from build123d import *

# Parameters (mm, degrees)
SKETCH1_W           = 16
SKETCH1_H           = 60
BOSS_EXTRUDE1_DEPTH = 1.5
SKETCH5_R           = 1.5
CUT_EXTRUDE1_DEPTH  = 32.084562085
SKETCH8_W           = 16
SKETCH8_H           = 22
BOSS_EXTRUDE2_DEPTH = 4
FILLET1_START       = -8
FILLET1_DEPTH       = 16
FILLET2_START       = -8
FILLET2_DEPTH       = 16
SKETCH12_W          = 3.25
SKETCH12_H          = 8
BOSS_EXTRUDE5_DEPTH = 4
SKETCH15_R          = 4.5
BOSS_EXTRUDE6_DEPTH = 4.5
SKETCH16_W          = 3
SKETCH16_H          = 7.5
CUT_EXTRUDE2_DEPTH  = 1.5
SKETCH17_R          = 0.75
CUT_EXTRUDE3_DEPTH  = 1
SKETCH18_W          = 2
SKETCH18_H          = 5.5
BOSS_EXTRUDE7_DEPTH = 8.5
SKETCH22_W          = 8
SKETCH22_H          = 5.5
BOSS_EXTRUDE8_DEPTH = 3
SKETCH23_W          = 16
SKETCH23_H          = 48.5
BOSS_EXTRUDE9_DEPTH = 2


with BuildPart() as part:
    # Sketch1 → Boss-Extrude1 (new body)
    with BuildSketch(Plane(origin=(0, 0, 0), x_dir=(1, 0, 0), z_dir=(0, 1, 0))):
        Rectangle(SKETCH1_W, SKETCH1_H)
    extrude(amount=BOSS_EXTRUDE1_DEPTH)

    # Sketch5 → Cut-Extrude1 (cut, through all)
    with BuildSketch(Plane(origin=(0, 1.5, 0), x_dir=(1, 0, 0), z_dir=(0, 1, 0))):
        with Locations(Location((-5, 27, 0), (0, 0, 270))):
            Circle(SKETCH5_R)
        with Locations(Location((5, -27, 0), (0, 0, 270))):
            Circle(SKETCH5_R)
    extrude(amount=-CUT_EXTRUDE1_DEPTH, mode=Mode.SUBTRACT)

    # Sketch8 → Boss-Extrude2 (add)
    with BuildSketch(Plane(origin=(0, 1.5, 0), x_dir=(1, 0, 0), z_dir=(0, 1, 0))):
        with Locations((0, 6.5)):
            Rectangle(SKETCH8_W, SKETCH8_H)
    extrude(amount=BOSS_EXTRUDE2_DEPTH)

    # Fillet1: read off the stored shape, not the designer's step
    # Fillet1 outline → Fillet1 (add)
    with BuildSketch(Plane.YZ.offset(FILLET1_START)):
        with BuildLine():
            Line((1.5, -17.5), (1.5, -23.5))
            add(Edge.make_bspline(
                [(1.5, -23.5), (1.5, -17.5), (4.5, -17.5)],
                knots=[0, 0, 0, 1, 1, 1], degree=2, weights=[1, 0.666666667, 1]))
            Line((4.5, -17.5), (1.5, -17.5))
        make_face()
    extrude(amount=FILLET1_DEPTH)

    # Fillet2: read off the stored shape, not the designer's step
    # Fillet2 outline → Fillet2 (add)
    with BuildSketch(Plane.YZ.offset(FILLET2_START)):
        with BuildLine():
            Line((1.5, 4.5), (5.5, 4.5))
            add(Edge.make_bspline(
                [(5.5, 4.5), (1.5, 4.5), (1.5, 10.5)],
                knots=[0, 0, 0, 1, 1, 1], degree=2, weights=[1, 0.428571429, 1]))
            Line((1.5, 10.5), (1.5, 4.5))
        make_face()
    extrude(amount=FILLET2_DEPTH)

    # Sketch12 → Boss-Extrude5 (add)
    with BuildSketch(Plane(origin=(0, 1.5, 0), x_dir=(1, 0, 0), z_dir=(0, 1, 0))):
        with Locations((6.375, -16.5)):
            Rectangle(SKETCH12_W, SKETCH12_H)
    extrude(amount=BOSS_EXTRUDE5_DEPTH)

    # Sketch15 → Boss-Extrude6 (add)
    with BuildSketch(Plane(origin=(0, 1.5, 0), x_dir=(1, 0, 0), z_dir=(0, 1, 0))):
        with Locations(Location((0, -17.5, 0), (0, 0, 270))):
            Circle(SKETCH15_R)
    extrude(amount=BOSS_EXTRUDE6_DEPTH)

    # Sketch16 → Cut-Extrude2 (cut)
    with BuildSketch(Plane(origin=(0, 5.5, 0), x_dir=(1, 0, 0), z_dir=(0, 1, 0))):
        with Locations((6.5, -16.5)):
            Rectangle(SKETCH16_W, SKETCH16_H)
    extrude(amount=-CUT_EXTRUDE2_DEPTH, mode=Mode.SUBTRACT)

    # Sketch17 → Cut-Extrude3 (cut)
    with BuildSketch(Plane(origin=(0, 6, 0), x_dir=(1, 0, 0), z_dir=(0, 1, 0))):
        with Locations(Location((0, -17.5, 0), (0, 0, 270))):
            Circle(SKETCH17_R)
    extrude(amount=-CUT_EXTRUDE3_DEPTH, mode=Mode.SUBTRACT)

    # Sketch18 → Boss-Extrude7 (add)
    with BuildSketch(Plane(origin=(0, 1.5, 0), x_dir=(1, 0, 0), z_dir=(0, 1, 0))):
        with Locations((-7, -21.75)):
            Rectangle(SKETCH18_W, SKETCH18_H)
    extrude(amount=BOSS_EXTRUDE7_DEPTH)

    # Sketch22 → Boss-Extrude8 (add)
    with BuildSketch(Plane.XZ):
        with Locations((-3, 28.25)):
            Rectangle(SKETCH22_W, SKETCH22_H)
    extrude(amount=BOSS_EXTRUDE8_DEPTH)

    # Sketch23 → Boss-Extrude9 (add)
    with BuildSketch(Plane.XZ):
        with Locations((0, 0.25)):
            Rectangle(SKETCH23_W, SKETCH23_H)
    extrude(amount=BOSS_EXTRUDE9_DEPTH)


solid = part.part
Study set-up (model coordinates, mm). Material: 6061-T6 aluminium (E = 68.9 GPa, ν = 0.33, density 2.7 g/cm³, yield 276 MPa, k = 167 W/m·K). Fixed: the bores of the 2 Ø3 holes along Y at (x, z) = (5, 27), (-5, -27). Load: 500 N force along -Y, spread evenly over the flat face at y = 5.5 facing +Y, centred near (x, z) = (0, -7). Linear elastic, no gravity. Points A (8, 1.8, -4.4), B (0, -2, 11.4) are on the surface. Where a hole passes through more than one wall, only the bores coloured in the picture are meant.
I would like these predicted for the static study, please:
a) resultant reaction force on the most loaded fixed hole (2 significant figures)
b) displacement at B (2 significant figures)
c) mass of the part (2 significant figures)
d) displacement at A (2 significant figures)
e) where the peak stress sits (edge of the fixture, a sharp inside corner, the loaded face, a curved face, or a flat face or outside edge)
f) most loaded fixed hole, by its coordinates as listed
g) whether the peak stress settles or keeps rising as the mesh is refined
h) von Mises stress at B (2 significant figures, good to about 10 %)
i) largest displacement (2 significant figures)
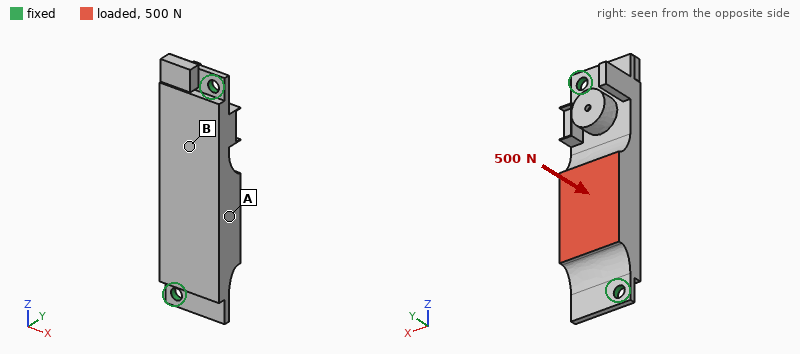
340 N
63 µm
14 g
88 µm
edge of the fixture
(-5, -27)
keeps rising
61 MPa
91 µm
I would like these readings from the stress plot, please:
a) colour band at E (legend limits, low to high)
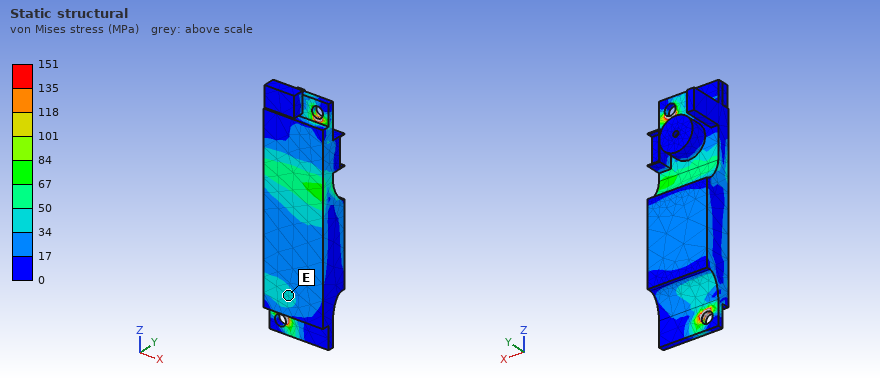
34 to 50 MPa
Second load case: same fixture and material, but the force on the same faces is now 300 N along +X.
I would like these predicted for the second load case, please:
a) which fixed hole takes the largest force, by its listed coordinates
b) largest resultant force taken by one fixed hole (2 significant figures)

(-5, -27)
190 N
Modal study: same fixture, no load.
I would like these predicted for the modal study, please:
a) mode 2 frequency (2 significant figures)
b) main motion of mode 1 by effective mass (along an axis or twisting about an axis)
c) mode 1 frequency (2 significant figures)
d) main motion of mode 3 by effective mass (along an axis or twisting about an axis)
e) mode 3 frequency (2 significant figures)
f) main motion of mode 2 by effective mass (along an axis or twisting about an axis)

4200 Hz
twisting about Z
4000 Hz
along X
9500 Hz
along Y
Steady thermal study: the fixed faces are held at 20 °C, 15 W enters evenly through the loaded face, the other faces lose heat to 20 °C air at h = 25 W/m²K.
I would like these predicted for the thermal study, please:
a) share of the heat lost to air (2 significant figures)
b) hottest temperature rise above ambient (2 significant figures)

6.2 %
21 K
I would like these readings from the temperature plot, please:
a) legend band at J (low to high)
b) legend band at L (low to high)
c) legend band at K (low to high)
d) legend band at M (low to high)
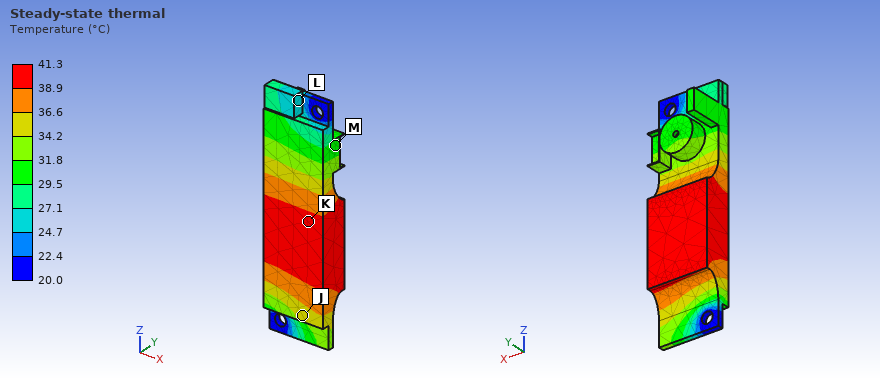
34.2 to 36.6 °C
24.7 to 27.1 °C
38.9 to 41.3 °C
29.5 to 31.8 °C
